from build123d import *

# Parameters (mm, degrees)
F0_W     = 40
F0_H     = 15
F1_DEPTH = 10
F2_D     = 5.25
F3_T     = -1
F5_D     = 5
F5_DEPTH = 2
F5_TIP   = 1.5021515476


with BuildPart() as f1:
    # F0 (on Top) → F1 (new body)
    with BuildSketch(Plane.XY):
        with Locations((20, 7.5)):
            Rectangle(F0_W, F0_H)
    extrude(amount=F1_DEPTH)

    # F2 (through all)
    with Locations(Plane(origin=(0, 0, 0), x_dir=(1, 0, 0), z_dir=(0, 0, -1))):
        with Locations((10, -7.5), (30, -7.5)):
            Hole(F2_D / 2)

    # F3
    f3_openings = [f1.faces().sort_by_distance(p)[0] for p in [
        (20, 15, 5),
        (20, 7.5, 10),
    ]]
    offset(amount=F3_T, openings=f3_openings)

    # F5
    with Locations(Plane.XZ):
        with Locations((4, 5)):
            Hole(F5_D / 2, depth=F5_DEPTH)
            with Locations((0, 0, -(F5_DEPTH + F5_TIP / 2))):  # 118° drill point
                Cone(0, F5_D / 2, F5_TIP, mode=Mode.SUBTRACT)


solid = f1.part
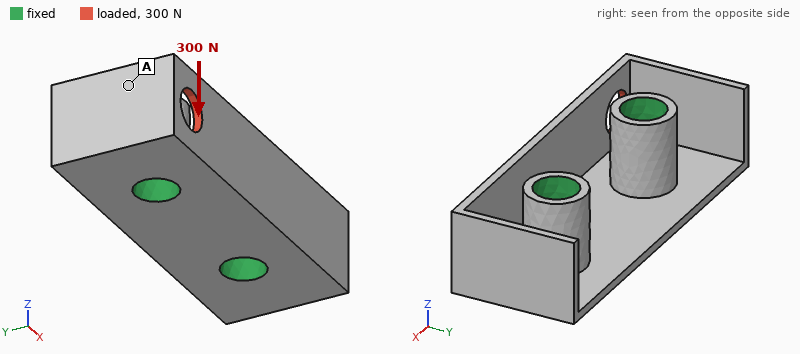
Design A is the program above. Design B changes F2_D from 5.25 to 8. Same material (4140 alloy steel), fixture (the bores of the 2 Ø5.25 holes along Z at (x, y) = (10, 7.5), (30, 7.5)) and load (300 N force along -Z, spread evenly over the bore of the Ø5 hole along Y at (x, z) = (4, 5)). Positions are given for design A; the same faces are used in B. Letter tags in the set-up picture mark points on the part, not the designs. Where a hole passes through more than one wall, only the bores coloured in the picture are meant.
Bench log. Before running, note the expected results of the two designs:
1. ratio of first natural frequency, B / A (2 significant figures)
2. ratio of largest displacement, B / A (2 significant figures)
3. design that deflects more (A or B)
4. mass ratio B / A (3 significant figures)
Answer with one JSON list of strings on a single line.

["1.2", "0.46", "A", "1.07"]
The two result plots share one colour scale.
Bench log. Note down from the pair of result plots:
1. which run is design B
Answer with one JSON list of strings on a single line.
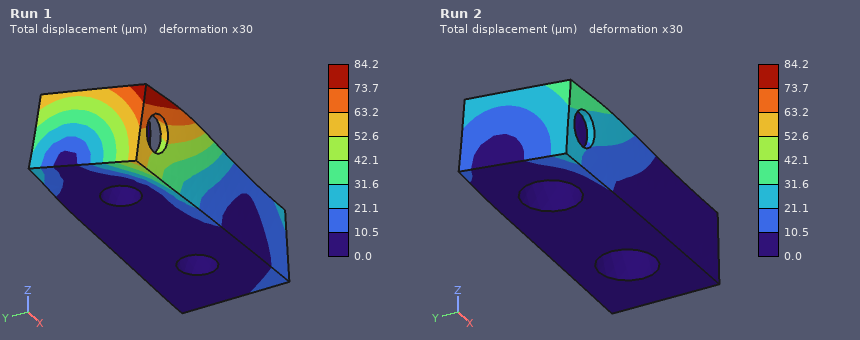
["Run 2"]
